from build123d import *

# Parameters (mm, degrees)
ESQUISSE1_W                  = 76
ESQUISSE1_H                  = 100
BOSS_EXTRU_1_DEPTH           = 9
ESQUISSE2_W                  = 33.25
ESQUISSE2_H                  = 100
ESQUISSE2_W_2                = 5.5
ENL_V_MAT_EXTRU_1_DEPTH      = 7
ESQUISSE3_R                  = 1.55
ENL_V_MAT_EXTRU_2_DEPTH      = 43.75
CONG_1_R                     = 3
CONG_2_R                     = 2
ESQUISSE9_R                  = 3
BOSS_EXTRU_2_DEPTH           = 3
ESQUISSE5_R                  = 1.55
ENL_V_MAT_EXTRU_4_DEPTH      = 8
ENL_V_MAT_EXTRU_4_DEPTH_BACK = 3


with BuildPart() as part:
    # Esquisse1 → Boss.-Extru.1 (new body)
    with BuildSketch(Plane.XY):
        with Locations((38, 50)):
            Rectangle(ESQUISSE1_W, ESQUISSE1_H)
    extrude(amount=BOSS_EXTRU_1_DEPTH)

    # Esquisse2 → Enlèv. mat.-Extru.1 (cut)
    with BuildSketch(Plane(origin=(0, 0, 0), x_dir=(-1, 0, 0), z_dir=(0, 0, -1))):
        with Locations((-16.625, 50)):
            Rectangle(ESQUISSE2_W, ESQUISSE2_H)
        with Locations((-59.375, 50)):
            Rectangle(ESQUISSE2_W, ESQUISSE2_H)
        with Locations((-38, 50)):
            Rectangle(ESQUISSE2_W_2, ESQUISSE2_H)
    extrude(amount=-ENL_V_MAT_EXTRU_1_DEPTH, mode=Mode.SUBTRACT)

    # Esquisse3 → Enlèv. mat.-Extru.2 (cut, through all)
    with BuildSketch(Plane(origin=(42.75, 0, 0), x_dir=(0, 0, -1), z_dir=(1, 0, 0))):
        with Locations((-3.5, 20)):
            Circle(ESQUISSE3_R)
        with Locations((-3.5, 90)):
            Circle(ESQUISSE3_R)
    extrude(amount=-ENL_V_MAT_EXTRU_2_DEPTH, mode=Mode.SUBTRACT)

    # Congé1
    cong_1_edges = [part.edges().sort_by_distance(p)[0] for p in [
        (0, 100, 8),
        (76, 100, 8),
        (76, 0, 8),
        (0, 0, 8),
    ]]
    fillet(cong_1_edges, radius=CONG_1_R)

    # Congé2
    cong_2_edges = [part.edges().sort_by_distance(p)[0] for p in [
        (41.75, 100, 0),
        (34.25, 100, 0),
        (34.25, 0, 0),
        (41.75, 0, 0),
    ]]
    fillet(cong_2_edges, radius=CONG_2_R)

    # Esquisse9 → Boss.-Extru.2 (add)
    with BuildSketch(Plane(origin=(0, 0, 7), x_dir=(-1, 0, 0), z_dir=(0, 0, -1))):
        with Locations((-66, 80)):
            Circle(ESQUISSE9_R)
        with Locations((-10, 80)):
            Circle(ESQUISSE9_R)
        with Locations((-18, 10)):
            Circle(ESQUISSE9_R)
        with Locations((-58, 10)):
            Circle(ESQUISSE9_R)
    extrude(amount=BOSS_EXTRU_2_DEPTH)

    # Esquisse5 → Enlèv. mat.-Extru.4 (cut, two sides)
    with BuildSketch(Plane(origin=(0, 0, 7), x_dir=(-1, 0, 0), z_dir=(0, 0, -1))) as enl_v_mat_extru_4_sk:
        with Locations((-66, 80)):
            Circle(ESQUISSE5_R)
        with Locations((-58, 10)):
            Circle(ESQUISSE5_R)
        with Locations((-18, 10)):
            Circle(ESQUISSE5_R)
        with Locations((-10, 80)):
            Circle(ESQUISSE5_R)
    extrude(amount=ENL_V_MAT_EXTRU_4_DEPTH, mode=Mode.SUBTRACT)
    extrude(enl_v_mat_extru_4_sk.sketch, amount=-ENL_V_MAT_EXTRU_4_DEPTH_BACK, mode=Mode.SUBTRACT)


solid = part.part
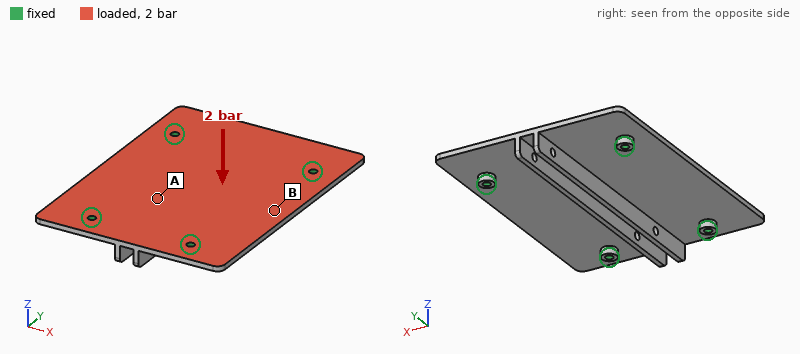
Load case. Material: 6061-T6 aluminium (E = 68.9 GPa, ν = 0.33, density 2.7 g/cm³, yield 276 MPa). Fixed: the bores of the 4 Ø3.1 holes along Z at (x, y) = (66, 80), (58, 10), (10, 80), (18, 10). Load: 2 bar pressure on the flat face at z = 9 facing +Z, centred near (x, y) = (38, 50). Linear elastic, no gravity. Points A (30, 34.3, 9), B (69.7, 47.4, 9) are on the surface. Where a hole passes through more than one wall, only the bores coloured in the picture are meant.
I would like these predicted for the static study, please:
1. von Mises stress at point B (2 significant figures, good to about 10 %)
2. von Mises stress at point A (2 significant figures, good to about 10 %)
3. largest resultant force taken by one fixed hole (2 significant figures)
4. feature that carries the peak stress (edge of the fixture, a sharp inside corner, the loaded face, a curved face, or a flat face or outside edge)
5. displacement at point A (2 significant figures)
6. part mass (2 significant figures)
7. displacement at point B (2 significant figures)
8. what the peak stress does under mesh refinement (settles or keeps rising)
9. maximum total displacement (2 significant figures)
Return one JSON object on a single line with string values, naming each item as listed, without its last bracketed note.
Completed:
{"von Mises stress at point B": "45 MPa", "von Mises stress at point A": "22 MPa", "largest resultant force taken by one fixed hole": "420 N", "feature that carries the peak stress": "edge of the fixture", "displacement at point A": "0.14 mm", "part mass": "49 g", "displacement at point B": "0.22 mm", "what the peak stress does under mesh refinement": "keeps rising", "maximum total displacement": "0.25 mm"}
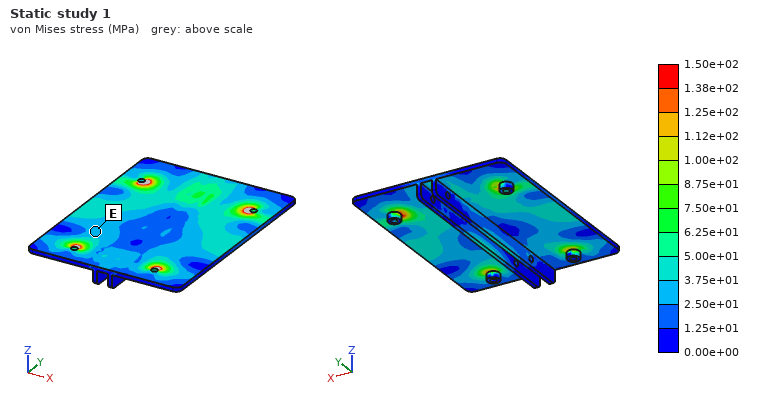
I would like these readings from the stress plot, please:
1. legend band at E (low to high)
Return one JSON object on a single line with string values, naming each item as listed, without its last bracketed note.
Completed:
{"legend band at E": "2.50e+01 to 3.75e+01 MPa"}
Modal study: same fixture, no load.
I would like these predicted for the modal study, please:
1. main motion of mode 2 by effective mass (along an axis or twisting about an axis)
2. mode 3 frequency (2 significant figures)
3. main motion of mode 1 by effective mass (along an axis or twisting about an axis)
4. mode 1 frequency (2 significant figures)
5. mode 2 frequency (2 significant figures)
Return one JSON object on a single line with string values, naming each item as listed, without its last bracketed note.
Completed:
{"main motion of mode 2 by effective mass": "twisting about Y", "mode 3 frequency": "2700 Hz", "main motion of mode 1 by effective mass": "along Z", "mode 1 frequency": "2200 Hz", "mode 2 frequency": "2400 Hz"}
